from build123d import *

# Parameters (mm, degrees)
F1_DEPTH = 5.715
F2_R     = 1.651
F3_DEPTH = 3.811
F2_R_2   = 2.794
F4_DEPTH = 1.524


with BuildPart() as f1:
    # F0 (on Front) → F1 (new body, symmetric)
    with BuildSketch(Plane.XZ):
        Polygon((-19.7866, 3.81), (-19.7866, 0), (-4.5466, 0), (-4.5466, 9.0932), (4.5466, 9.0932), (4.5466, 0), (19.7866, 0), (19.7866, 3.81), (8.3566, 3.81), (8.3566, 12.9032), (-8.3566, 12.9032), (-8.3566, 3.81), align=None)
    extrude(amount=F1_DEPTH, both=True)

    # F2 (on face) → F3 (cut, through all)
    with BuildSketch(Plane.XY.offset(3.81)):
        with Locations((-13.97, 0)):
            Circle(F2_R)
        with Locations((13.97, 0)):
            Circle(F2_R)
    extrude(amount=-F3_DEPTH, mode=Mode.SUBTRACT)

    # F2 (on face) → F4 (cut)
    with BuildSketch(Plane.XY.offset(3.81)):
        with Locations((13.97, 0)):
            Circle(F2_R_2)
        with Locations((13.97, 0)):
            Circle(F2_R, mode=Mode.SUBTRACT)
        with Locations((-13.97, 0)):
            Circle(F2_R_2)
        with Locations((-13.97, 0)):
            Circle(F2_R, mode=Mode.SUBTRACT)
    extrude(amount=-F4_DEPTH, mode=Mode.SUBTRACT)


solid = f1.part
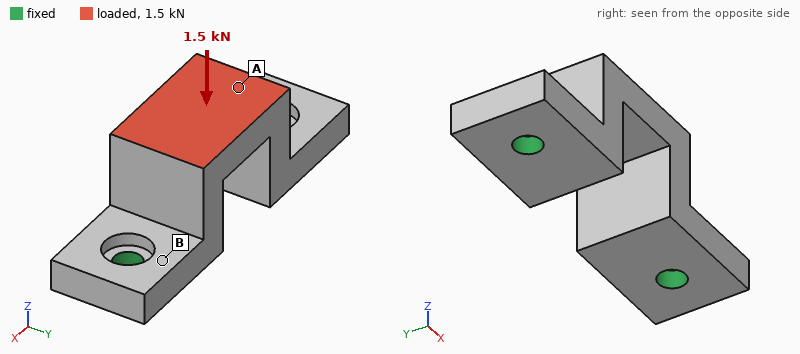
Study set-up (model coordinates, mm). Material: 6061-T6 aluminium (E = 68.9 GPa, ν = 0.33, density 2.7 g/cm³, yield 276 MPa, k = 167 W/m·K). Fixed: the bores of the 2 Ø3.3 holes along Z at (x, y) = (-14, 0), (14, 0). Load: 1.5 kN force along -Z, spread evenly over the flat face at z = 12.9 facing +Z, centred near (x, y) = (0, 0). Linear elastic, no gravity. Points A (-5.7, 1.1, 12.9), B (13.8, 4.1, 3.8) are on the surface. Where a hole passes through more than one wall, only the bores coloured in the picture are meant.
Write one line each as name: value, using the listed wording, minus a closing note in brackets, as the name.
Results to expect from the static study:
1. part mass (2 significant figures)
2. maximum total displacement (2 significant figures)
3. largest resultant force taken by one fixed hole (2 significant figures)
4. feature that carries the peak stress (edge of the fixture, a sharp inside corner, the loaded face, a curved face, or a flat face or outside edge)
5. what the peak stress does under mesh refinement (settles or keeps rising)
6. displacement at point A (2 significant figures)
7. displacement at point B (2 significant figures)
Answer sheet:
part mass: 6.5 g
maximum total displacement: 21 µm
largest resultant force taken by one fixed hole: 890 N
feature that carries the peak stress: edge of the fixture
what the peak stress does under mesh refinement: keeps rising
displacement at point A: 20 µm
displacement at point B: 4.9 µm
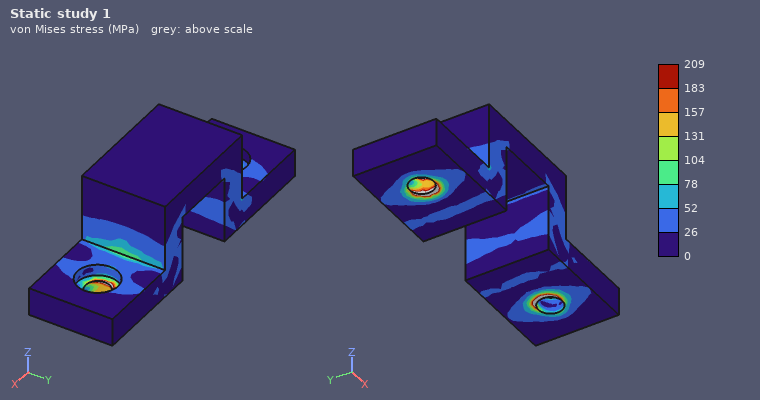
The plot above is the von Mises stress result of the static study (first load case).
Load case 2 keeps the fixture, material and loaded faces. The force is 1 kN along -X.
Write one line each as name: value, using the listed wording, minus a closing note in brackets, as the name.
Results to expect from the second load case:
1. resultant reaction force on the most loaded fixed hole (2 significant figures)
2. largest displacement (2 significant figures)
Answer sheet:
resultant reaction force on the most loaded fixed hole: 690 N
largest displacement: 22 µm
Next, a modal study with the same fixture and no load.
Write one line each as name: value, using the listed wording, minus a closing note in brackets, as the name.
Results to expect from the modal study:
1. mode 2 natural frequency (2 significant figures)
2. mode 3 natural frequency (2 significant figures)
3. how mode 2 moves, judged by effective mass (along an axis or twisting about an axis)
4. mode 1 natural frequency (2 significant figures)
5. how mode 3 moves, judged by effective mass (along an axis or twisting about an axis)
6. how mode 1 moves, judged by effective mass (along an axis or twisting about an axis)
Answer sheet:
mode 2 natural frequency: 21 kHz
mode 3 natural frequency: 23 kHz
how mode 2 moves, judged by effective mass: along Z
mode 1 natural frequency: 9100 Hz
how mode 3 moves, judged by effective mass: along X
how mode 1 moves, judged by effective mass: along Y
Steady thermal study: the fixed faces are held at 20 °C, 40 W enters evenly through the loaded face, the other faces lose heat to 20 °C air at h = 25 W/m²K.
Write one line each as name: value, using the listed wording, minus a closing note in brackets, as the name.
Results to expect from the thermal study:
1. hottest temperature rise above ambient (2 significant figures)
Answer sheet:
hottest temperature rise above ambient: 49 K
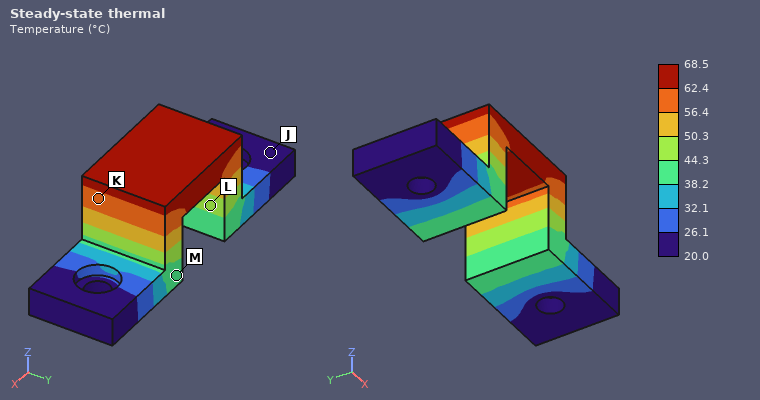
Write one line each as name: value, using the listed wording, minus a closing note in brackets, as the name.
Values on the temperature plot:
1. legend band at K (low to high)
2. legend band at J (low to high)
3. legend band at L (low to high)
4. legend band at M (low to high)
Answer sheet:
legend band at K: 56.4 to 62.4 °C
legend band at J: 20.0 to 26.1 °C
legend band at L: 44.3 to 50.3 °C
legend band at M: 38.2 to 44.3 °C
